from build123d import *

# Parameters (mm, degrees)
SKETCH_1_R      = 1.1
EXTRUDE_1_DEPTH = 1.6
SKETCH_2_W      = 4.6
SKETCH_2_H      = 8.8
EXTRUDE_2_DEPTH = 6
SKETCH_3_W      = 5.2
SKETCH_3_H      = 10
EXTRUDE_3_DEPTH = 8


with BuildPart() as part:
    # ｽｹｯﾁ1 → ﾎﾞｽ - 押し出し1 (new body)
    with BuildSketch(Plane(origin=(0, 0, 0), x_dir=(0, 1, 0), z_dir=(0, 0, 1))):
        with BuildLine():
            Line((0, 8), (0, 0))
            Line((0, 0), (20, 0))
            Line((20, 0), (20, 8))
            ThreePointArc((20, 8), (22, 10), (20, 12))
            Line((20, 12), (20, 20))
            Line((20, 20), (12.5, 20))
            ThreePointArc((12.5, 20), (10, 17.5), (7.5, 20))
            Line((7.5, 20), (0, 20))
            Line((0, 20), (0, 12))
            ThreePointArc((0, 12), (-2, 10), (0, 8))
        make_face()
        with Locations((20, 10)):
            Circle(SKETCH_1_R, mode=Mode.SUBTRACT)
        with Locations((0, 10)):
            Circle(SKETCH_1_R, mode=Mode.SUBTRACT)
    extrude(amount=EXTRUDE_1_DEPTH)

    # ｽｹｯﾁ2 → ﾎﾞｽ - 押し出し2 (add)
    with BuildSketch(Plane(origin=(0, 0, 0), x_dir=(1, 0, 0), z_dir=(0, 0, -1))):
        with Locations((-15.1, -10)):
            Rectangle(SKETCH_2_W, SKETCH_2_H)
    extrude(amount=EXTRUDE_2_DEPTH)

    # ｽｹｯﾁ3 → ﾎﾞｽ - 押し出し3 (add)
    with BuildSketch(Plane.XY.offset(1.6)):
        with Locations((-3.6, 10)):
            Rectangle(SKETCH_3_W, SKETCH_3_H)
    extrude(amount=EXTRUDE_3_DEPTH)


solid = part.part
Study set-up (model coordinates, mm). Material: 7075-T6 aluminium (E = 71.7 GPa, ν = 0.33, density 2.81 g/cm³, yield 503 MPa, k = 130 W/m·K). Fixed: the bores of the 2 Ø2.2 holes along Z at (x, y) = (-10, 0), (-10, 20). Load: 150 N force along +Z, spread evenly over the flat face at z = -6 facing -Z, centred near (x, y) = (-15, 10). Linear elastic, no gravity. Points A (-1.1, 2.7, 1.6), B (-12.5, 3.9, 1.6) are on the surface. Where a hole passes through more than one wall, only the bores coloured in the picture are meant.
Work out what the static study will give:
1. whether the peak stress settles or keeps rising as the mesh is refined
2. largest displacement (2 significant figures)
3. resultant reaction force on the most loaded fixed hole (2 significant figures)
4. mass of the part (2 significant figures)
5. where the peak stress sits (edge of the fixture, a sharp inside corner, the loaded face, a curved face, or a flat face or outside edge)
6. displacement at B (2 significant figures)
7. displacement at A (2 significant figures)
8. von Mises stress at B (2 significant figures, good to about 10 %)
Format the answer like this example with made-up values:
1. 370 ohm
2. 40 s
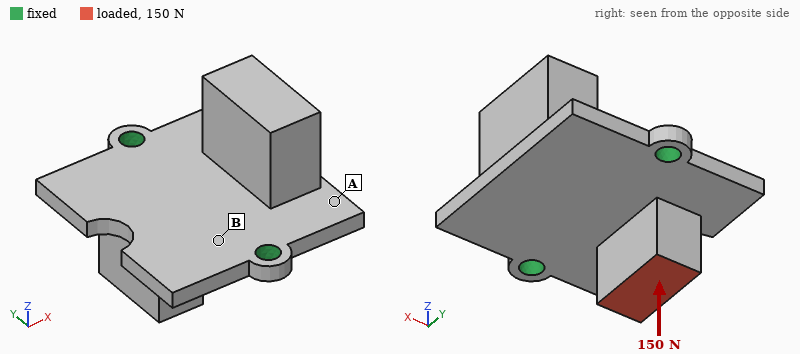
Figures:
1. keeps rising
2. 67 µm
3. 77 N
4. 3.6 g
5. edge of the fixture
6. 15 µm
7. 20 µm
8. 50 MPa
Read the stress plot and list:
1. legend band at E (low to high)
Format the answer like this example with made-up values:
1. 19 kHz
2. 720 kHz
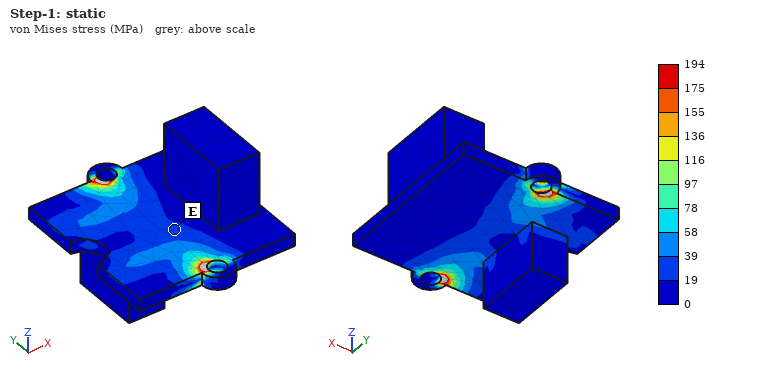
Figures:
1. 19 to 39 MPa
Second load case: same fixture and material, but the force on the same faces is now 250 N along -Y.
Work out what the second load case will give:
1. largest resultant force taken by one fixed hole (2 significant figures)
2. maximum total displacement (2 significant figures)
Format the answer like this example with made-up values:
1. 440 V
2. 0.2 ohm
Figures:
1. 180 N
2. 30 µm
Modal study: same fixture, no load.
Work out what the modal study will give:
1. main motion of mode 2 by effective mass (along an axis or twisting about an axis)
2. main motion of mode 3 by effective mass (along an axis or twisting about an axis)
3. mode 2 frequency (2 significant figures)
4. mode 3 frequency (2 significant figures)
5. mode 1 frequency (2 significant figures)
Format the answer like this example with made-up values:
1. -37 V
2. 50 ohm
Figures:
1. along Z
2. along Y
3. 8300 Hz
4. 15 kHz
5. 4800 Hz
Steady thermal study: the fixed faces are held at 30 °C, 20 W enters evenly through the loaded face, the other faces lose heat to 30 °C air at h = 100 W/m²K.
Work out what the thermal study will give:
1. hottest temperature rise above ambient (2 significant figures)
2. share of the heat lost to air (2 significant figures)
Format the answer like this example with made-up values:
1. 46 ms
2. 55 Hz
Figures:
1. 63 K
2. 15 %
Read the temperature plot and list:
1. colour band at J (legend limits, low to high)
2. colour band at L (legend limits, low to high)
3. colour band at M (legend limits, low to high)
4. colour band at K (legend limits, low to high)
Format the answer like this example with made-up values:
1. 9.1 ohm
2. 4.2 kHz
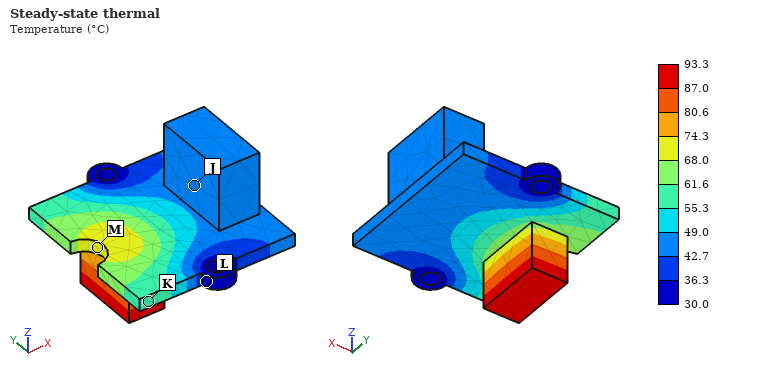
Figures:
1. 42.7 to 49.0 °C
2. 30.0 to 36.3 °C
3. 68.0 to 74.3 °C
4. 55.3 to 61.6 °C
